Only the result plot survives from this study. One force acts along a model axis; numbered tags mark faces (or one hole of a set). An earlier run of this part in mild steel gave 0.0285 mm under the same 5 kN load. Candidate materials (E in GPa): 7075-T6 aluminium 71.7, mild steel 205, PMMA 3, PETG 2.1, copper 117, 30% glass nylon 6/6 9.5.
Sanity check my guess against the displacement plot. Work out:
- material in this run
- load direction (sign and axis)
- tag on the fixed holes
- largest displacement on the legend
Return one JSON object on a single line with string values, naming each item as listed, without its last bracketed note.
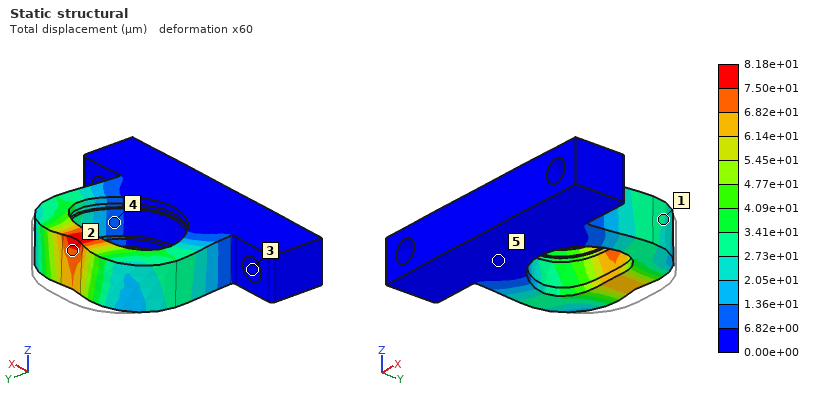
{"material in this run": "7075-T6 aluminium", "load direction": "-Y", "tag on the fixed holes": "3", "largest displacement on the legend": "8.18e+01 µm"}
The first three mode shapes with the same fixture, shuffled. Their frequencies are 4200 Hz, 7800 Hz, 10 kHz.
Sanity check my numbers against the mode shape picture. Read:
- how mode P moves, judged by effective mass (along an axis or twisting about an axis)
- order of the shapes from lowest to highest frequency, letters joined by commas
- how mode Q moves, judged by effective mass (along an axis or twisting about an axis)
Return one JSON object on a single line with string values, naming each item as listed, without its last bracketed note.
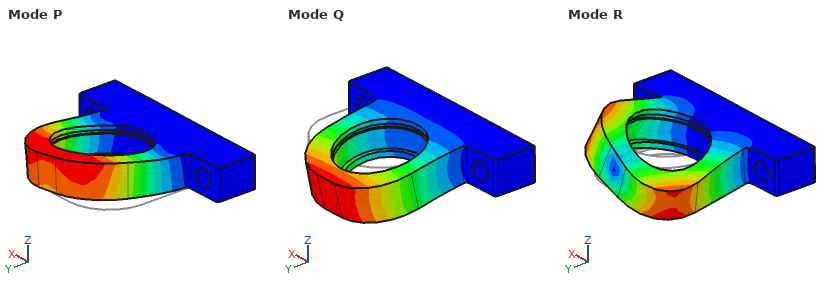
{"how mode P moves, judged by effective mass": "along X", "order of the shapes from lowest to highest frequency, letters joined by commas": "Q, P, R", "how mode Q moves, judged by effective mass": "along Z"}
